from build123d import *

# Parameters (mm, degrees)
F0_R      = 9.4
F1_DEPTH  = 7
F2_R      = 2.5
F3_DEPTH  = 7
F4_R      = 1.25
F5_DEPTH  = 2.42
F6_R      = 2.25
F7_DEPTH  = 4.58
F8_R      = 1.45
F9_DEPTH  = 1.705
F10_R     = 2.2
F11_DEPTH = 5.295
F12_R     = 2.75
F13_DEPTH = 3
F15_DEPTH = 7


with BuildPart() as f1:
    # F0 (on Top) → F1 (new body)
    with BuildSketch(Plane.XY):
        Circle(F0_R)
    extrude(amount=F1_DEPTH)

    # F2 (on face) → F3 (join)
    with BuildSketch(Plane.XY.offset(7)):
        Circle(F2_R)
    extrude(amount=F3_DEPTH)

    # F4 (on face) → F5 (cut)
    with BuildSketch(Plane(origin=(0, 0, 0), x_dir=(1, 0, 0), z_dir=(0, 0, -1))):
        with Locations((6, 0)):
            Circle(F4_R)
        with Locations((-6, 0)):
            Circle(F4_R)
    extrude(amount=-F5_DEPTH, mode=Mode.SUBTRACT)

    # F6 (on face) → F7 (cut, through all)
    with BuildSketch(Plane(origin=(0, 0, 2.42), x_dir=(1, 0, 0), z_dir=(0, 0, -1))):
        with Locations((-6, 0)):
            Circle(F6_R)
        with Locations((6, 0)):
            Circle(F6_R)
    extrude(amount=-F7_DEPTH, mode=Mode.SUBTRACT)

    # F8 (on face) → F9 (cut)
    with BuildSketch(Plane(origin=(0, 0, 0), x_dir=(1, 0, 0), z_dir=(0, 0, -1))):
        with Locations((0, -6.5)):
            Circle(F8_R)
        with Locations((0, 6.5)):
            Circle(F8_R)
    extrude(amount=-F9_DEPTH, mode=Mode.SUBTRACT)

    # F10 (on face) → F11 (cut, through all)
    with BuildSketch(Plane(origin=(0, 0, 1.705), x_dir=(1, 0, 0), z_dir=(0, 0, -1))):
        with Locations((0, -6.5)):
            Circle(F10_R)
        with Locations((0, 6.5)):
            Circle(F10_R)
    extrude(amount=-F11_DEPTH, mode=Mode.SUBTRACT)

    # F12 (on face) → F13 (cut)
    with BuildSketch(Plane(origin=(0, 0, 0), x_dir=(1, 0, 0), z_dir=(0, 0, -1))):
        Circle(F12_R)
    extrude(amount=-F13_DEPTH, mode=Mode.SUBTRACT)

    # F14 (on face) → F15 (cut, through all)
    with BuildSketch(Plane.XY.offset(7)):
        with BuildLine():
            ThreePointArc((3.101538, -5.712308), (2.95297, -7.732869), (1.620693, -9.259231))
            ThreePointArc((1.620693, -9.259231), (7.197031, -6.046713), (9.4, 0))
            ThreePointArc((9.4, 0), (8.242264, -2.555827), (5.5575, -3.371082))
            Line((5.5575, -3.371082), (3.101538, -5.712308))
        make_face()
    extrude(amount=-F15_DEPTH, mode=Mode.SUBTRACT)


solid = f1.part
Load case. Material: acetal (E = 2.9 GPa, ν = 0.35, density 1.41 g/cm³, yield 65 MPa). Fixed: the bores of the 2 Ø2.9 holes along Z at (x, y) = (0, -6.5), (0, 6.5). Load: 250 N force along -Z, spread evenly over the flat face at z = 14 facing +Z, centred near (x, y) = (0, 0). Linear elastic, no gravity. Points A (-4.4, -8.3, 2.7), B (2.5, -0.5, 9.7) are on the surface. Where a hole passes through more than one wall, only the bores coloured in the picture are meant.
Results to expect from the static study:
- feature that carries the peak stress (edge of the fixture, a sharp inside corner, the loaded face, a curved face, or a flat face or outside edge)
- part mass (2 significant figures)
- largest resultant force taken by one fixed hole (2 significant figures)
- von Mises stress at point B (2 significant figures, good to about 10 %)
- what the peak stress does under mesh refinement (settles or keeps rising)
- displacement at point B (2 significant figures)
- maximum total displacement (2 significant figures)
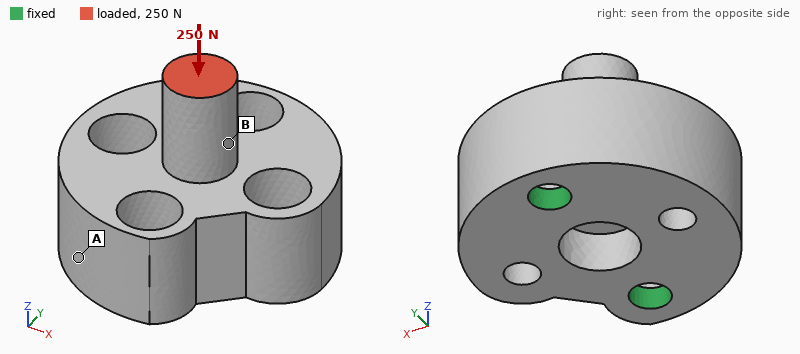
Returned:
edge of the fixture
2.1 g
140 N
13 MPa
keeps rising
46 µm
65 µm
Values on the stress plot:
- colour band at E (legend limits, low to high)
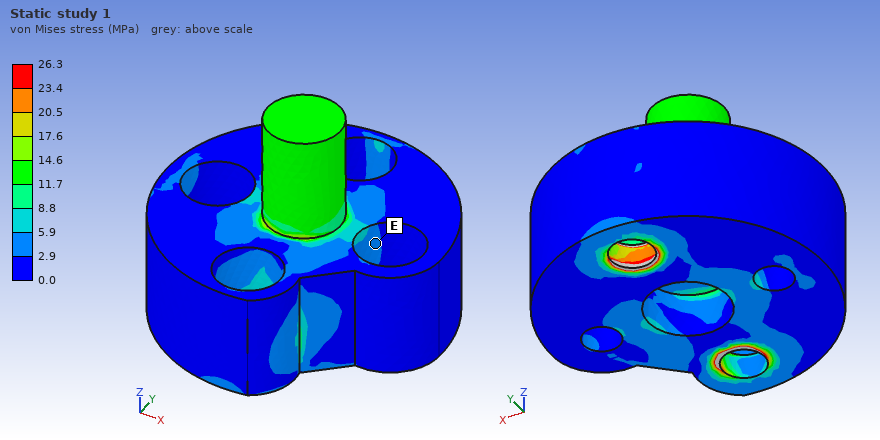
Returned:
2.9 to 5.9 MPa
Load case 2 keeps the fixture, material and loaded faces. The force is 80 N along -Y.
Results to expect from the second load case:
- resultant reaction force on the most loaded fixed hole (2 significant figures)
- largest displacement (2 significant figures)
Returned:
92 N
0.23 mm
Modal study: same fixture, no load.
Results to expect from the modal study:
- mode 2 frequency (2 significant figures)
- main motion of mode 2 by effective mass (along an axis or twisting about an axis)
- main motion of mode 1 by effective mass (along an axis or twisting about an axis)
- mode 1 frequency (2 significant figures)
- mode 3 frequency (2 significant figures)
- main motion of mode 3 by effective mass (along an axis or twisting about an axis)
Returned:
11 kHz
along Y
along X
3900 Hz
11 kHz
along Z
